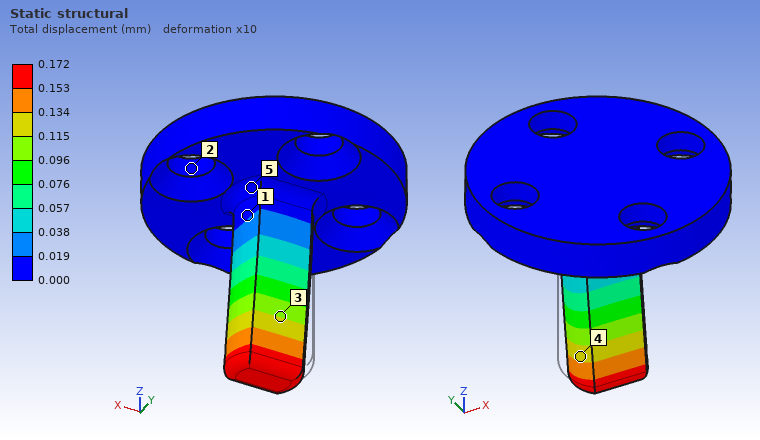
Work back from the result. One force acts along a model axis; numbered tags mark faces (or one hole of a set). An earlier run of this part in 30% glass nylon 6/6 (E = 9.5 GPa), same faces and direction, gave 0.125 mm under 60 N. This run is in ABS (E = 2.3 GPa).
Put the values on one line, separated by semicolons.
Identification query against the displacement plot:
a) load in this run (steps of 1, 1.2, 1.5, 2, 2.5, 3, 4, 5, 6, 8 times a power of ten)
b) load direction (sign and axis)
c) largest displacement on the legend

20 N; -Y; 0.172 mm
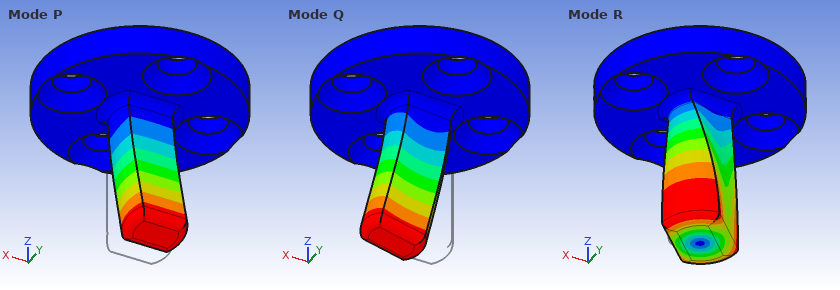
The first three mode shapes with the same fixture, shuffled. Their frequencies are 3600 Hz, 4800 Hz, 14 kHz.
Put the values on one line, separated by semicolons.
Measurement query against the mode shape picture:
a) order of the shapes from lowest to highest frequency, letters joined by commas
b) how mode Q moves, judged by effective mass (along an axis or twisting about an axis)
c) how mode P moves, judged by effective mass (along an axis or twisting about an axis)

P, Q, R; along X; along Y
